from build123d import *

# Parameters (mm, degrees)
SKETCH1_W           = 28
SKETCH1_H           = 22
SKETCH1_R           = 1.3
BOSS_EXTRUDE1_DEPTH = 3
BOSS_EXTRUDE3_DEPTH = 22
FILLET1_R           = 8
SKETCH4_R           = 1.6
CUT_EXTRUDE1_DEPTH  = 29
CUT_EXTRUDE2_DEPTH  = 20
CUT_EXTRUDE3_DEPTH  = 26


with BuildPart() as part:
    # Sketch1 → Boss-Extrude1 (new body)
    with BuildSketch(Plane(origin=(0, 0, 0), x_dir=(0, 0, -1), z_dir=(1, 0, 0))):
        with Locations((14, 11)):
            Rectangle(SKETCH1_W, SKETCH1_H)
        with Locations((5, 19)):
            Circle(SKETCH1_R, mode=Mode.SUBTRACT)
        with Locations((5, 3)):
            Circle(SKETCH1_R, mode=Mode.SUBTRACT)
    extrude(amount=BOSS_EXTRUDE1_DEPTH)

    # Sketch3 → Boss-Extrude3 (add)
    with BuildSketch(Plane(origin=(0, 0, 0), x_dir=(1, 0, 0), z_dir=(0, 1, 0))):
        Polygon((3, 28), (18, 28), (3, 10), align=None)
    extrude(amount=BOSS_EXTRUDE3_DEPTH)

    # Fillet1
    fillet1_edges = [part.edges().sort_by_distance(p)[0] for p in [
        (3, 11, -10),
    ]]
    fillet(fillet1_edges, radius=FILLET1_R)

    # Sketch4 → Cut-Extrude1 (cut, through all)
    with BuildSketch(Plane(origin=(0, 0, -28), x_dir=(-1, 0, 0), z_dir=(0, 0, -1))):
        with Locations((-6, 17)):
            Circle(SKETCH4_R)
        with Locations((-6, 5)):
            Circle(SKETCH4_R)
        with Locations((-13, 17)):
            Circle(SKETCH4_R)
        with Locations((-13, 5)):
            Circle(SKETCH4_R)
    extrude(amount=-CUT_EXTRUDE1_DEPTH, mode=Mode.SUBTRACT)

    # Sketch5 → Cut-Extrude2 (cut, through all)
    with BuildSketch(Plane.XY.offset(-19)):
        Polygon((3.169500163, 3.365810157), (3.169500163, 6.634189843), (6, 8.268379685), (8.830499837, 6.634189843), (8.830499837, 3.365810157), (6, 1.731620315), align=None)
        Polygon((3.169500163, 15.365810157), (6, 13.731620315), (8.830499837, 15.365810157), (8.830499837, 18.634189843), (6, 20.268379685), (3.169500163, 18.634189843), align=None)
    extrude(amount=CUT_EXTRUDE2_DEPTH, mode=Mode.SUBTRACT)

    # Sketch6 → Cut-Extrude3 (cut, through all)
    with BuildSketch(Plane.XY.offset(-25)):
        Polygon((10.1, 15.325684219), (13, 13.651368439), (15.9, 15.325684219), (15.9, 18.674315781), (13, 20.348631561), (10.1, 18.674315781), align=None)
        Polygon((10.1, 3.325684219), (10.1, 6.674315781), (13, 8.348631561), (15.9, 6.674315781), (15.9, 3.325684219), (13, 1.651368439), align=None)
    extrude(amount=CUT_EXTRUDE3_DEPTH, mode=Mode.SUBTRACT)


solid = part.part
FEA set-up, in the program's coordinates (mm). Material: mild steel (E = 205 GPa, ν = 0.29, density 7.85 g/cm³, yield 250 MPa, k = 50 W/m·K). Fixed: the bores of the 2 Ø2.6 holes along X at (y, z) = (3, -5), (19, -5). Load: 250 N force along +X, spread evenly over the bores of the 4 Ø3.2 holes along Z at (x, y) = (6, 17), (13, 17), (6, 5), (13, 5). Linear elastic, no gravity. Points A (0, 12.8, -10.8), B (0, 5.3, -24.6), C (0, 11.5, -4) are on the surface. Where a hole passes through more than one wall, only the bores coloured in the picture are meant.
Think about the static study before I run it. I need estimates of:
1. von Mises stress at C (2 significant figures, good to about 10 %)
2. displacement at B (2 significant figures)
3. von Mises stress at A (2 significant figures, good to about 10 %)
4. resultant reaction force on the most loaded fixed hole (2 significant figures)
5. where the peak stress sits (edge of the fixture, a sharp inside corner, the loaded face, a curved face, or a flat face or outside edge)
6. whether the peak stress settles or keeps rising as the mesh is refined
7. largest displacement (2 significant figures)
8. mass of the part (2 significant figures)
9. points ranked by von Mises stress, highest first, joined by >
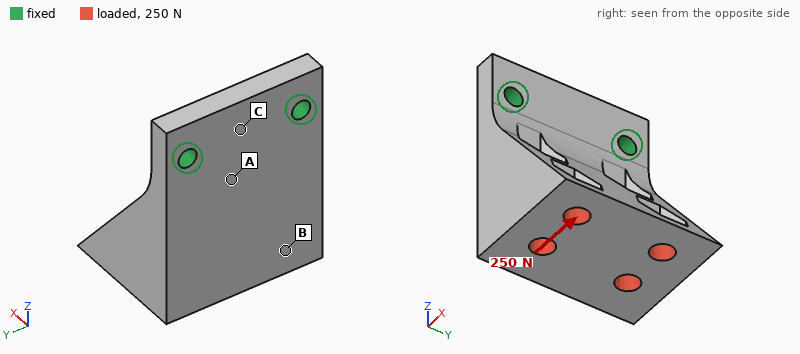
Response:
32 MPa
44 µm
62 MPa
130 N
edge of the fixture
keeps rising
69 µm
32 g
A > C > B
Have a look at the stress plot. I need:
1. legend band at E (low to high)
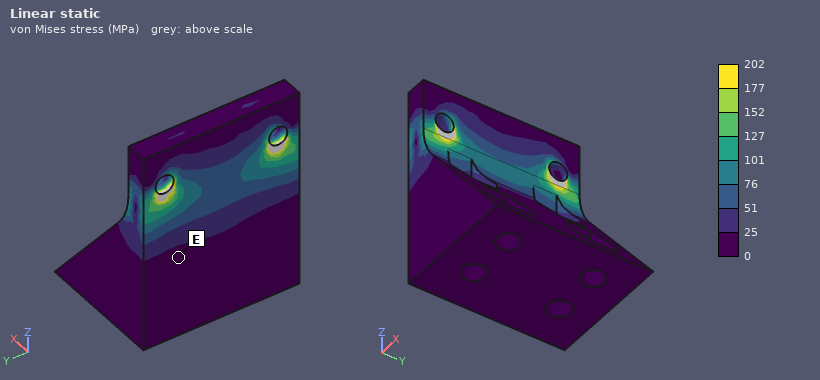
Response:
0 to 25 MPa
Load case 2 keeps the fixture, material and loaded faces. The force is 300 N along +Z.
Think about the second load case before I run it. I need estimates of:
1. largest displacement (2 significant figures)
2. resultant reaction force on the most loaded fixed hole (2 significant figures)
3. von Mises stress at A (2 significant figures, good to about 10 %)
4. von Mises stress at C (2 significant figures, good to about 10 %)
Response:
32 µm
150 N
30 MPa
14 MPa
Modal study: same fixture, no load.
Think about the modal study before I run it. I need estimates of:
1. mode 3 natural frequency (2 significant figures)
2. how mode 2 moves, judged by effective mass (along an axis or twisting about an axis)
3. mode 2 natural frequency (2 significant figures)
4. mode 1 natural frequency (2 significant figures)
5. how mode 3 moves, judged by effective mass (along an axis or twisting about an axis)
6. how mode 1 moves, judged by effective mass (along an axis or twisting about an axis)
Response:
14 kHz
along Y
8600 Hz
2400 Hz
along Y
along X
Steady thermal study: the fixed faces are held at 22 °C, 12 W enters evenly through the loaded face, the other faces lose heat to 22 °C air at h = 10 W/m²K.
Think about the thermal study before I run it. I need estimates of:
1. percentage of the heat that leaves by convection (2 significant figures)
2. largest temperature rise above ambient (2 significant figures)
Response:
6.9 %
51 K
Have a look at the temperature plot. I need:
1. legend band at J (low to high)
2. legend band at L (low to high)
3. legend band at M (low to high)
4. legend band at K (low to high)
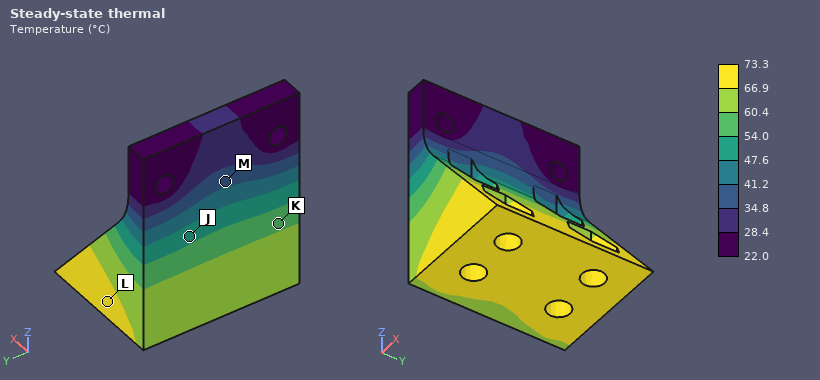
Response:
47.6 to 54.0 °C
66.9 to 73.3 °C
34.8 to 41.2 °C
54.0 to 60.4 °C
